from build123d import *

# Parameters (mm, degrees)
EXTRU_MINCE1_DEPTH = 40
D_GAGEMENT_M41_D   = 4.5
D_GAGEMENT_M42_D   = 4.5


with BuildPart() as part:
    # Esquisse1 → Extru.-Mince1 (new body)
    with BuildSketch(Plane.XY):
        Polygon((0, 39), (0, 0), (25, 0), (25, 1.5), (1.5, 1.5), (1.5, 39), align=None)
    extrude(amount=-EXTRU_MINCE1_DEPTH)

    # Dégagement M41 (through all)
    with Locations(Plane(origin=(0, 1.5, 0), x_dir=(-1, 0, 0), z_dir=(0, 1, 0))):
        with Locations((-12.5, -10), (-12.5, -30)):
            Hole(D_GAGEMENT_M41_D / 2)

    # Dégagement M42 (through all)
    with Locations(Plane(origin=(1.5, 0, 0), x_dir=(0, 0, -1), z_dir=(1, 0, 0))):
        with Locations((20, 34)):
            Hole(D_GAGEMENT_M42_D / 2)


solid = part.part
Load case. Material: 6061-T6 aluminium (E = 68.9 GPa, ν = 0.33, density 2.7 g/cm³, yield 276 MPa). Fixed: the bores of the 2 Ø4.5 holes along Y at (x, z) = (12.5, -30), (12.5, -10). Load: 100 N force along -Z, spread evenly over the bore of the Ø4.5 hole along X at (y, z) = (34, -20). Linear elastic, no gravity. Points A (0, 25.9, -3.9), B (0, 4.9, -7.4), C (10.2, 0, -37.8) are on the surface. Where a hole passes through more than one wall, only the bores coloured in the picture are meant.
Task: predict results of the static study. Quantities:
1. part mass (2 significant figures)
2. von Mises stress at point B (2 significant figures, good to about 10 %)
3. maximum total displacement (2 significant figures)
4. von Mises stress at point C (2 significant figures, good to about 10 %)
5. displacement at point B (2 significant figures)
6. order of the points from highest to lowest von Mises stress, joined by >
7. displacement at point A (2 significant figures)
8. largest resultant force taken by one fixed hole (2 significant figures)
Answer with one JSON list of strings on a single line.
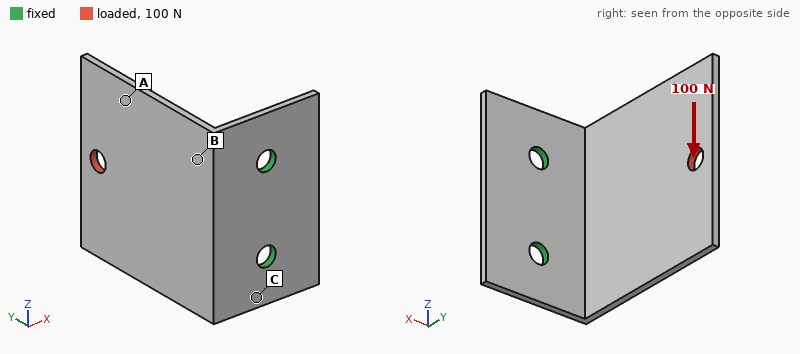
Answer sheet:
["9.9 g", "40 MPa", "0.36 mm", "74 MPa", "0.11 mm", "C > B > A", "0.24 mm", "150 N"]
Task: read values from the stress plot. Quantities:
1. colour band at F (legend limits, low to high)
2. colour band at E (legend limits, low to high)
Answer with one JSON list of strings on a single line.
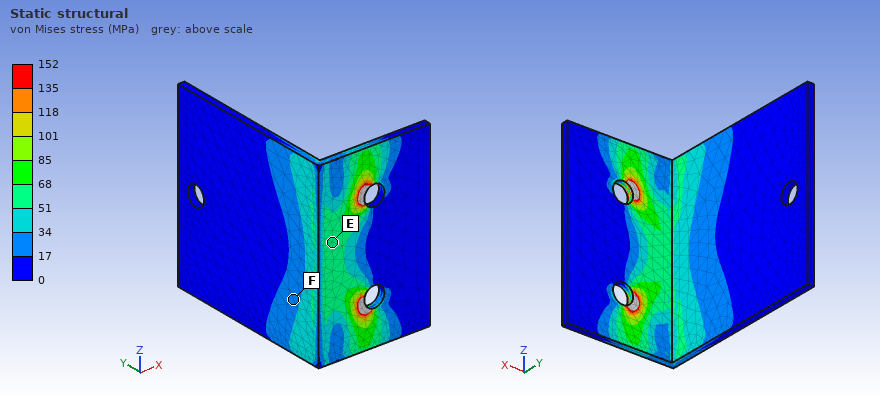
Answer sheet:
["17 to 34 MPa", "51 to 68 MPa"]
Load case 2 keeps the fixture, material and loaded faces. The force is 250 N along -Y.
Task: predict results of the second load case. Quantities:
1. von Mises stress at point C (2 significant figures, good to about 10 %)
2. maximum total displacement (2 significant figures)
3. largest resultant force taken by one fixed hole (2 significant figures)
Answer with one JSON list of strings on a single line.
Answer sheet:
["81 MPa", "0.70 mm", "130 N"]
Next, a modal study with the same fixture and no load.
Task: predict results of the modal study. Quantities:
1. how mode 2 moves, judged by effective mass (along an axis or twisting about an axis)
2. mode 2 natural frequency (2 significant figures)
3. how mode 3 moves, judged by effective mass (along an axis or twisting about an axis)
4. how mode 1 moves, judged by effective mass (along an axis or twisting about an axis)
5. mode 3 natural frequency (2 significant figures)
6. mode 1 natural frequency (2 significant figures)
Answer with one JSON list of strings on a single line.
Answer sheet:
["along Z", "1500 Hz", "along Z", "along X", "2100 Hz", "600 Hz"]
